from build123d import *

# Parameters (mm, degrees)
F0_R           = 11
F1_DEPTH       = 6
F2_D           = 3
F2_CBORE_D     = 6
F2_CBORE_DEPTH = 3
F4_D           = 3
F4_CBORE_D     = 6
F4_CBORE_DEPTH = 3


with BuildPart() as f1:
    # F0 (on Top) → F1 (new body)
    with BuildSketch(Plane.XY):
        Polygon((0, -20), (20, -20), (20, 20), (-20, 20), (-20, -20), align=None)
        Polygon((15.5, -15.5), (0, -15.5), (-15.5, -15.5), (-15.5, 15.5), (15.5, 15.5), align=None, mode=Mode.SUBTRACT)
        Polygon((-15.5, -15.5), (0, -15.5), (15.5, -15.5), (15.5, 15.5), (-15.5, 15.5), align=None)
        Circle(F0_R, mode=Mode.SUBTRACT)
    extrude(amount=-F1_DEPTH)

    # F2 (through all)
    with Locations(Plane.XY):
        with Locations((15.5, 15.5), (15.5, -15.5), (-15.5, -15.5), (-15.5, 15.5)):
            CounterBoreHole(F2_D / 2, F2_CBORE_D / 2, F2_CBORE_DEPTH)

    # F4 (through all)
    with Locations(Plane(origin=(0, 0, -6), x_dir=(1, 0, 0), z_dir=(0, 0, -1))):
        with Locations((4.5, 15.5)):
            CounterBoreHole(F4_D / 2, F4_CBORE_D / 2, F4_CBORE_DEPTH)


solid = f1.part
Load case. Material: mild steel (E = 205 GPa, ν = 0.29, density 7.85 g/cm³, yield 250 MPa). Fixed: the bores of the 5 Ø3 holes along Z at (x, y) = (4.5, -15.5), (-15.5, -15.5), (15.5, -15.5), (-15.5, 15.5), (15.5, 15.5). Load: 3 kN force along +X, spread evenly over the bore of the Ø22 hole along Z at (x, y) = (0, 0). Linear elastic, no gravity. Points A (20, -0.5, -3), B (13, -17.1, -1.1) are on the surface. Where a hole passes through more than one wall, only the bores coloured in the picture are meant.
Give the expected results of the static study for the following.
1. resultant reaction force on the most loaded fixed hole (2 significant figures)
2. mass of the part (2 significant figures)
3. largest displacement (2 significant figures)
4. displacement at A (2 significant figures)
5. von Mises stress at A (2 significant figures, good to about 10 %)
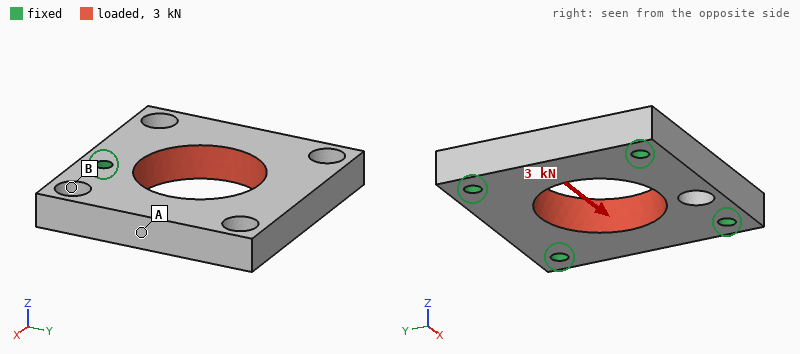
750 N
53 g
2.4 µm
1.7 µm
16 MPa
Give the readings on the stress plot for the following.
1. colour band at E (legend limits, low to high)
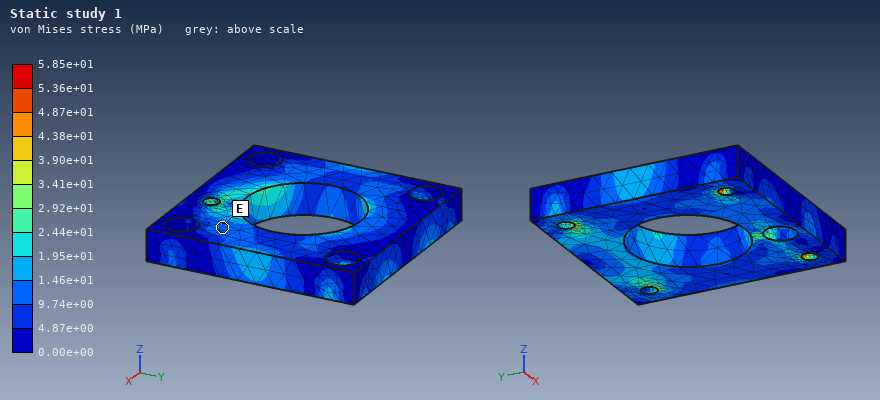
9.74e+00 to 1.46e+01 MPa
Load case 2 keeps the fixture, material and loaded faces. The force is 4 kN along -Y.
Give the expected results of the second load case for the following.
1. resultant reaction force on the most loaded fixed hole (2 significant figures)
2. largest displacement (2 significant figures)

940 N
3.6 µm
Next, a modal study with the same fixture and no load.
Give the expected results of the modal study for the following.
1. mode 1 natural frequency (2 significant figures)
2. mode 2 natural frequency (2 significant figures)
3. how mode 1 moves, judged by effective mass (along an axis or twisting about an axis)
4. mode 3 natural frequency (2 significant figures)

20 kHz
22 kHz
along Z
23 kHz
